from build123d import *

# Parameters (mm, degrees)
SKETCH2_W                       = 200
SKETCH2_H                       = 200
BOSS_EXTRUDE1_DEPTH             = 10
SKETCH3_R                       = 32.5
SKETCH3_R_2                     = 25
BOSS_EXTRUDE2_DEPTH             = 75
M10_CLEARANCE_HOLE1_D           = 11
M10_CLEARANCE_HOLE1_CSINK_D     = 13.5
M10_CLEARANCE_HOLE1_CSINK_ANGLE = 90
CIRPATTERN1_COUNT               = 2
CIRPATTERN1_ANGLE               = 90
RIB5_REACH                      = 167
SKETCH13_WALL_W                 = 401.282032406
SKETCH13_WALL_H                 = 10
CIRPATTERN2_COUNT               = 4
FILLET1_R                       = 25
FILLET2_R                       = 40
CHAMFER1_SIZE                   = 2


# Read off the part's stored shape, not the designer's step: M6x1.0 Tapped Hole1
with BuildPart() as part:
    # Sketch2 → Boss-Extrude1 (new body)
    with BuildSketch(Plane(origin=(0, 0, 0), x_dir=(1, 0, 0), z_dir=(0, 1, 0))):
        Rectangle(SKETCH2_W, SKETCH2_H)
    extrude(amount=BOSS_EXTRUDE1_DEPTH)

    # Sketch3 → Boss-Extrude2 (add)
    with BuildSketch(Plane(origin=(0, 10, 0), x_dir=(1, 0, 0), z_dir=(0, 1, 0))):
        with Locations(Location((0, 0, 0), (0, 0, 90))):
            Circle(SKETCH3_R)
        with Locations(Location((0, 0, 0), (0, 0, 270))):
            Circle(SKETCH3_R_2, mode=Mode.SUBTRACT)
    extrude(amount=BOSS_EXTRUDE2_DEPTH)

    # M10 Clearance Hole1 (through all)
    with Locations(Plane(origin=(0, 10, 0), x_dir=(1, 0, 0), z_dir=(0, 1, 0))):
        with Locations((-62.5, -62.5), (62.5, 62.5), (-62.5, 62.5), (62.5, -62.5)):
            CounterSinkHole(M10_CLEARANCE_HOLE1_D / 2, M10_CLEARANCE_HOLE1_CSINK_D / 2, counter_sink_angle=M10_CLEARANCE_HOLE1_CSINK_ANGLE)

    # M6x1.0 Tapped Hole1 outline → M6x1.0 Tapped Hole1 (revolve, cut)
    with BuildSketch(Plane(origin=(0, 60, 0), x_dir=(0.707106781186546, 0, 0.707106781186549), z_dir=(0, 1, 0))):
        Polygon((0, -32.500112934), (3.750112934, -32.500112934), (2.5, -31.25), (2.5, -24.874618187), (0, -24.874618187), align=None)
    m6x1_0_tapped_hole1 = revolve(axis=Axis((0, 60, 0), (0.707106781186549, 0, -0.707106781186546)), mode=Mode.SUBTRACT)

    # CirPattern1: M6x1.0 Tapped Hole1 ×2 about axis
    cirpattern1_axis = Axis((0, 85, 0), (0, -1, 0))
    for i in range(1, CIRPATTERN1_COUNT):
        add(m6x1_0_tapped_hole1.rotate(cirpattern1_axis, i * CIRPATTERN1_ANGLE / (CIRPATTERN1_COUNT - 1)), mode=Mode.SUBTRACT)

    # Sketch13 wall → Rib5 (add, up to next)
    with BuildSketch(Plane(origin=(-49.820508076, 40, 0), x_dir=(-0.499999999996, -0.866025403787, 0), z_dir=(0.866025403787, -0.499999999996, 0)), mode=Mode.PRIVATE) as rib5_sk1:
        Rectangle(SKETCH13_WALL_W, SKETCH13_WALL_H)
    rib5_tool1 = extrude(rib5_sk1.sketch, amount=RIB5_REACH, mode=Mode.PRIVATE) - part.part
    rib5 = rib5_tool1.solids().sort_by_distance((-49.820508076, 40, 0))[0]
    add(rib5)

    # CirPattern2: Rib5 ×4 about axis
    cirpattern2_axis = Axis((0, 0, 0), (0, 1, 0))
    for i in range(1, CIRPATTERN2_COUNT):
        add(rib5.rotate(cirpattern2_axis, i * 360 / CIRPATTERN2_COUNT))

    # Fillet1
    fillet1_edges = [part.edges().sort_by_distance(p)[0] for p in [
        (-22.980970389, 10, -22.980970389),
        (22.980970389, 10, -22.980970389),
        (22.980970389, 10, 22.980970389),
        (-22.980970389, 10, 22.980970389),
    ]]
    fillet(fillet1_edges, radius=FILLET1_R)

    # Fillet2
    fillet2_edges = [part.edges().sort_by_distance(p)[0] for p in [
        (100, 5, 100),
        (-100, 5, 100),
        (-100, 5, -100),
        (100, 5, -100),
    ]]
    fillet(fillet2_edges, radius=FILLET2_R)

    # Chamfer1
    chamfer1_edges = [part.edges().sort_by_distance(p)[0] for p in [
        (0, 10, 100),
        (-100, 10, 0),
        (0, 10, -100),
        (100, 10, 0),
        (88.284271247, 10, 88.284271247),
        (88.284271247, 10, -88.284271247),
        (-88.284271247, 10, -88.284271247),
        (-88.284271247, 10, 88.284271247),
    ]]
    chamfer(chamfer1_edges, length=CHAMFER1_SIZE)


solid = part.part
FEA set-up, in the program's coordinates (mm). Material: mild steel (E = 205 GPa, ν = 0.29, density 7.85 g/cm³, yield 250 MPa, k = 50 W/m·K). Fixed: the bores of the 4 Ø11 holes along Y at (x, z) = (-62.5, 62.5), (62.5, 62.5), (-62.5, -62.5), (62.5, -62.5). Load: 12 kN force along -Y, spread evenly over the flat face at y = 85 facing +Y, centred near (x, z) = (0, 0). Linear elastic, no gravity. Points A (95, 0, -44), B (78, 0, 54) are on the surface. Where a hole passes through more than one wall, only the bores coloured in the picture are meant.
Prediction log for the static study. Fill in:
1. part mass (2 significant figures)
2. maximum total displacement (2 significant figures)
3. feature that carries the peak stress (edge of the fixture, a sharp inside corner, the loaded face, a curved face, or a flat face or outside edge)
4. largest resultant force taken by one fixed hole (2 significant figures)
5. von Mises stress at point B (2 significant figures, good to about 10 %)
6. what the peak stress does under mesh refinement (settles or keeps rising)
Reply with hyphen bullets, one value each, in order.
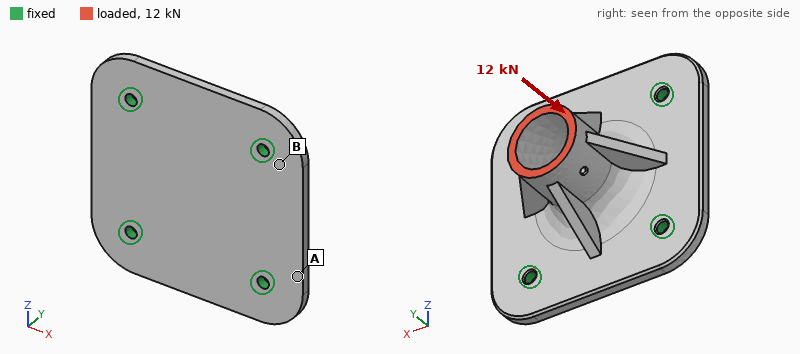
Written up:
- 4.3 kg
- 28 µm
- edge of the fixture
- 3.4 kN
- 15 MPa
- keeps rising
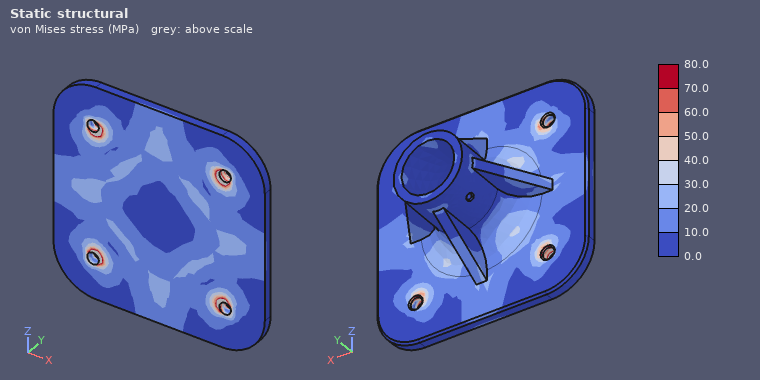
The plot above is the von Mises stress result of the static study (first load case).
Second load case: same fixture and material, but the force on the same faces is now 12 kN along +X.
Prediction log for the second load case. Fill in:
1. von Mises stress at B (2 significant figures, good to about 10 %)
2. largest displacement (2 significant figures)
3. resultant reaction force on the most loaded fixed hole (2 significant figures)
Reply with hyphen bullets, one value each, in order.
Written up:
- 31 MPa
- 84 µm
- 5.4 kN
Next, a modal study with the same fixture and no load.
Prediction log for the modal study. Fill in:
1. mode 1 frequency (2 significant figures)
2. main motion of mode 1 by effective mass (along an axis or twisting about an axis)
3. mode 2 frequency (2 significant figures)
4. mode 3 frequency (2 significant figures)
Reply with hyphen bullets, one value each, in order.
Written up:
- 2100 Hz
- along Y
- 2500 Hz
- 2500 Hz
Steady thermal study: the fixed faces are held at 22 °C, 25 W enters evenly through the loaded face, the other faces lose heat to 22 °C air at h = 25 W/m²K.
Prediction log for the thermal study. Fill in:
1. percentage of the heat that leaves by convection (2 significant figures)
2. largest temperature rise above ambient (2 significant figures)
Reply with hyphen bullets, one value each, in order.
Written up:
- 53 %
- 22 K
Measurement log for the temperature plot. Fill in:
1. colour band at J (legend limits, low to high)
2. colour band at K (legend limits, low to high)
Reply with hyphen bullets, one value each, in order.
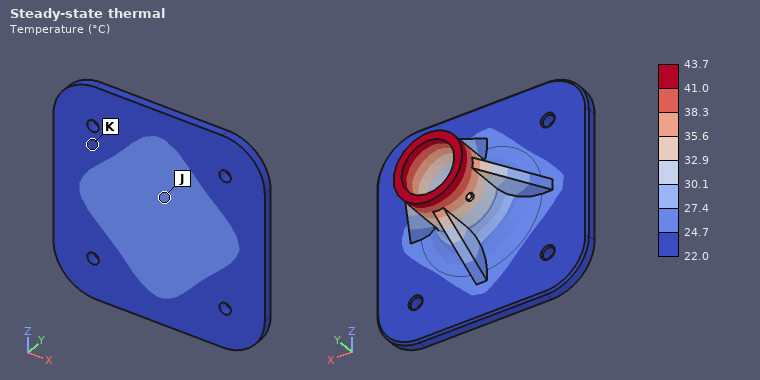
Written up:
- 24.7 to 27.4 °C
- 22.0 to 24.7 °C
